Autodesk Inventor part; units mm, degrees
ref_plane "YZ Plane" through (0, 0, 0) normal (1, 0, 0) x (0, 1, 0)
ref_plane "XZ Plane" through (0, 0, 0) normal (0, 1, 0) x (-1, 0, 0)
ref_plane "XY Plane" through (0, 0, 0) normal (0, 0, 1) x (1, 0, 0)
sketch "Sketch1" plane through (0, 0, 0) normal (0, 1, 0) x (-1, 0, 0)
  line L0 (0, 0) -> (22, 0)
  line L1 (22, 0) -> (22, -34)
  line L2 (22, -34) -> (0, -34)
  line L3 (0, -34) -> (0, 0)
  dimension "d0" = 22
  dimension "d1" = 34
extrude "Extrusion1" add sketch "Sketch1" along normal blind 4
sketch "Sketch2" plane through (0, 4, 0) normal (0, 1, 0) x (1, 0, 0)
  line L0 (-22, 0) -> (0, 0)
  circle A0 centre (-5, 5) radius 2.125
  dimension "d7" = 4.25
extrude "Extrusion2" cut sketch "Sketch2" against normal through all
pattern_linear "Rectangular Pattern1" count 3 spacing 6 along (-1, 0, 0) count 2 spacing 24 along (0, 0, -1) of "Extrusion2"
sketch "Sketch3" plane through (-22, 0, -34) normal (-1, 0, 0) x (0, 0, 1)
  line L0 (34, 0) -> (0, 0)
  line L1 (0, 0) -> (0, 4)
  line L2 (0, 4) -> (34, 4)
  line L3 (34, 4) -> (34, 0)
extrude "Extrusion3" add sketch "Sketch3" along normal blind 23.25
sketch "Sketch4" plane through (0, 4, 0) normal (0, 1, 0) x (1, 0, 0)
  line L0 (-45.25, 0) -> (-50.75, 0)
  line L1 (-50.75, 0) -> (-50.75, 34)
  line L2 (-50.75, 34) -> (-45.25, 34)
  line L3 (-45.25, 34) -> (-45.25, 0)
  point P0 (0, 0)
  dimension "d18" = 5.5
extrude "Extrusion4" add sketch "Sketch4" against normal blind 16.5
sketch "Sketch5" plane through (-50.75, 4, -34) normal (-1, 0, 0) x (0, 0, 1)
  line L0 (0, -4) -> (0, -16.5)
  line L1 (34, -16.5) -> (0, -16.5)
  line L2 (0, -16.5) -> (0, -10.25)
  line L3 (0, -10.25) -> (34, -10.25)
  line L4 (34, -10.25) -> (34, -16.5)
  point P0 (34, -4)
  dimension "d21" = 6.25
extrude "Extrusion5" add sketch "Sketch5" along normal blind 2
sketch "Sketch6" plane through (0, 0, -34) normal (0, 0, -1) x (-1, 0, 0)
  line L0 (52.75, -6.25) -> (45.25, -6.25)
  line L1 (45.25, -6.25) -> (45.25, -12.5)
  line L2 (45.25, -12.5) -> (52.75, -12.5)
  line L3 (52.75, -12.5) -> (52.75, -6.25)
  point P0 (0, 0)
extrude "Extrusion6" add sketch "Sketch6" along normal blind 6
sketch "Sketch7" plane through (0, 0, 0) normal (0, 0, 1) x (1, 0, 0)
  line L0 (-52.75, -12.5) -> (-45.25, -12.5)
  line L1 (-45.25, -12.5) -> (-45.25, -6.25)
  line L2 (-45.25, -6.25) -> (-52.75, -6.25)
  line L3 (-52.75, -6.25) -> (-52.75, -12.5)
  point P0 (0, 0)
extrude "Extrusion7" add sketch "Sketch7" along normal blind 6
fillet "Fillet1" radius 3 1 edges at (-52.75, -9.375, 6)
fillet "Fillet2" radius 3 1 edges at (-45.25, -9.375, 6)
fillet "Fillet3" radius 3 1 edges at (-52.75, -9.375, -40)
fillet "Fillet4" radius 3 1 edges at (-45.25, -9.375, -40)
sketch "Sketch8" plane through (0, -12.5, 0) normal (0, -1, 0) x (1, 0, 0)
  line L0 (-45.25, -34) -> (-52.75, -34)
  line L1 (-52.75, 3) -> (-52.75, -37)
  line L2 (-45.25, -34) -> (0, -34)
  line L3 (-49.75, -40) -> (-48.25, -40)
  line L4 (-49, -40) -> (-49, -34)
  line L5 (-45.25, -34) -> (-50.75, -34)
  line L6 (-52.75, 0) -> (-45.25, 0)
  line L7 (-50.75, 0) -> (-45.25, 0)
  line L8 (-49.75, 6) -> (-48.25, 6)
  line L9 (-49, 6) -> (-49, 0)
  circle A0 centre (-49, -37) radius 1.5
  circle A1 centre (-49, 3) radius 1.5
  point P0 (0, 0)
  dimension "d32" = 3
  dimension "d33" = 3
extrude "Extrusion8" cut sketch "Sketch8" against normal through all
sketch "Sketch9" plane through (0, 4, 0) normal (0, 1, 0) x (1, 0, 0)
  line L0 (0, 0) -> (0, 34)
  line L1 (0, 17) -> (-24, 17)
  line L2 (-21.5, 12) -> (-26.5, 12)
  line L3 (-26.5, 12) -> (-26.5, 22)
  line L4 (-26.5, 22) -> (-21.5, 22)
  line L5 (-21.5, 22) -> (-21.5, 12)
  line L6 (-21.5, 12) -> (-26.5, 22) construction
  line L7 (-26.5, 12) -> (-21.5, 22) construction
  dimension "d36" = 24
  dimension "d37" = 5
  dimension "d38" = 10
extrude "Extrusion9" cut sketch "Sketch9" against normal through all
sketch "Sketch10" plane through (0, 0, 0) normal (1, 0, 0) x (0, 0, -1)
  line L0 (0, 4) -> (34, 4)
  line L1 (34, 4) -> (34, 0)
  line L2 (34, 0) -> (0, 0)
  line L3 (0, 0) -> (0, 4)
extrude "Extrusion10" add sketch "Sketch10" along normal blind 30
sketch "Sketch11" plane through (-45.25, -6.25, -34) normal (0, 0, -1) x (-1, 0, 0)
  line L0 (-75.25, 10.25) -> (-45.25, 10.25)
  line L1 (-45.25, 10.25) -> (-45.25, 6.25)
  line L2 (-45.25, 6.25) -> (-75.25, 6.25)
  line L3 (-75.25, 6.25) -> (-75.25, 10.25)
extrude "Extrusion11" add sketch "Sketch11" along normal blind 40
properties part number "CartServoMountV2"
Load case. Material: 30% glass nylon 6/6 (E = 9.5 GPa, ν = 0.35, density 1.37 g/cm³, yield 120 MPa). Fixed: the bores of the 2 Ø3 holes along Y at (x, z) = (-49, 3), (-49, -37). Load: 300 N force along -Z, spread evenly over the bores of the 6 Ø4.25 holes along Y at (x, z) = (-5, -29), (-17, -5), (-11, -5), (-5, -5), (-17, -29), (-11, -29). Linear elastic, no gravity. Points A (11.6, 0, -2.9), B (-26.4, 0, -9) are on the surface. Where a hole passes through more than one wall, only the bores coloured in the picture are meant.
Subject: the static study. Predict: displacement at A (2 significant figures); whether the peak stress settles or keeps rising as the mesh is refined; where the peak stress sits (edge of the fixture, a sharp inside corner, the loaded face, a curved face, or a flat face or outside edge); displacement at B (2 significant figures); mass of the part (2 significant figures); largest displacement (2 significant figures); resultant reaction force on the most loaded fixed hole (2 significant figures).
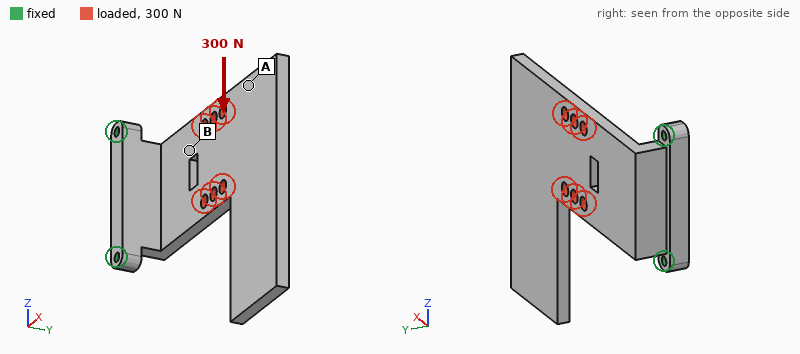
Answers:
0.67 mm
keeps rising
edge of the fixture
0.25 mm
25 g
1.1 mm
380 N
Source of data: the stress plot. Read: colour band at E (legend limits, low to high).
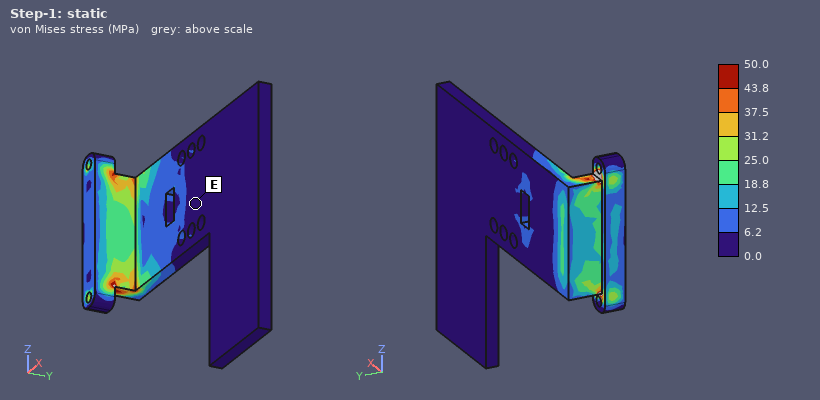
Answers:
0.0 to 6.2 MPa
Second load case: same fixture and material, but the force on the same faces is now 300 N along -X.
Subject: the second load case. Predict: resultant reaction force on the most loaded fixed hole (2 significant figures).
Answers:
150 N
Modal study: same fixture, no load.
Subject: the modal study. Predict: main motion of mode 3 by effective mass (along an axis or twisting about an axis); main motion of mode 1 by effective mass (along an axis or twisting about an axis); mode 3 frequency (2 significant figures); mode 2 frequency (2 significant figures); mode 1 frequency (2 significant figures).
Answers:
along Z
along Y
610 Hz
400 Hz
150 Hz
